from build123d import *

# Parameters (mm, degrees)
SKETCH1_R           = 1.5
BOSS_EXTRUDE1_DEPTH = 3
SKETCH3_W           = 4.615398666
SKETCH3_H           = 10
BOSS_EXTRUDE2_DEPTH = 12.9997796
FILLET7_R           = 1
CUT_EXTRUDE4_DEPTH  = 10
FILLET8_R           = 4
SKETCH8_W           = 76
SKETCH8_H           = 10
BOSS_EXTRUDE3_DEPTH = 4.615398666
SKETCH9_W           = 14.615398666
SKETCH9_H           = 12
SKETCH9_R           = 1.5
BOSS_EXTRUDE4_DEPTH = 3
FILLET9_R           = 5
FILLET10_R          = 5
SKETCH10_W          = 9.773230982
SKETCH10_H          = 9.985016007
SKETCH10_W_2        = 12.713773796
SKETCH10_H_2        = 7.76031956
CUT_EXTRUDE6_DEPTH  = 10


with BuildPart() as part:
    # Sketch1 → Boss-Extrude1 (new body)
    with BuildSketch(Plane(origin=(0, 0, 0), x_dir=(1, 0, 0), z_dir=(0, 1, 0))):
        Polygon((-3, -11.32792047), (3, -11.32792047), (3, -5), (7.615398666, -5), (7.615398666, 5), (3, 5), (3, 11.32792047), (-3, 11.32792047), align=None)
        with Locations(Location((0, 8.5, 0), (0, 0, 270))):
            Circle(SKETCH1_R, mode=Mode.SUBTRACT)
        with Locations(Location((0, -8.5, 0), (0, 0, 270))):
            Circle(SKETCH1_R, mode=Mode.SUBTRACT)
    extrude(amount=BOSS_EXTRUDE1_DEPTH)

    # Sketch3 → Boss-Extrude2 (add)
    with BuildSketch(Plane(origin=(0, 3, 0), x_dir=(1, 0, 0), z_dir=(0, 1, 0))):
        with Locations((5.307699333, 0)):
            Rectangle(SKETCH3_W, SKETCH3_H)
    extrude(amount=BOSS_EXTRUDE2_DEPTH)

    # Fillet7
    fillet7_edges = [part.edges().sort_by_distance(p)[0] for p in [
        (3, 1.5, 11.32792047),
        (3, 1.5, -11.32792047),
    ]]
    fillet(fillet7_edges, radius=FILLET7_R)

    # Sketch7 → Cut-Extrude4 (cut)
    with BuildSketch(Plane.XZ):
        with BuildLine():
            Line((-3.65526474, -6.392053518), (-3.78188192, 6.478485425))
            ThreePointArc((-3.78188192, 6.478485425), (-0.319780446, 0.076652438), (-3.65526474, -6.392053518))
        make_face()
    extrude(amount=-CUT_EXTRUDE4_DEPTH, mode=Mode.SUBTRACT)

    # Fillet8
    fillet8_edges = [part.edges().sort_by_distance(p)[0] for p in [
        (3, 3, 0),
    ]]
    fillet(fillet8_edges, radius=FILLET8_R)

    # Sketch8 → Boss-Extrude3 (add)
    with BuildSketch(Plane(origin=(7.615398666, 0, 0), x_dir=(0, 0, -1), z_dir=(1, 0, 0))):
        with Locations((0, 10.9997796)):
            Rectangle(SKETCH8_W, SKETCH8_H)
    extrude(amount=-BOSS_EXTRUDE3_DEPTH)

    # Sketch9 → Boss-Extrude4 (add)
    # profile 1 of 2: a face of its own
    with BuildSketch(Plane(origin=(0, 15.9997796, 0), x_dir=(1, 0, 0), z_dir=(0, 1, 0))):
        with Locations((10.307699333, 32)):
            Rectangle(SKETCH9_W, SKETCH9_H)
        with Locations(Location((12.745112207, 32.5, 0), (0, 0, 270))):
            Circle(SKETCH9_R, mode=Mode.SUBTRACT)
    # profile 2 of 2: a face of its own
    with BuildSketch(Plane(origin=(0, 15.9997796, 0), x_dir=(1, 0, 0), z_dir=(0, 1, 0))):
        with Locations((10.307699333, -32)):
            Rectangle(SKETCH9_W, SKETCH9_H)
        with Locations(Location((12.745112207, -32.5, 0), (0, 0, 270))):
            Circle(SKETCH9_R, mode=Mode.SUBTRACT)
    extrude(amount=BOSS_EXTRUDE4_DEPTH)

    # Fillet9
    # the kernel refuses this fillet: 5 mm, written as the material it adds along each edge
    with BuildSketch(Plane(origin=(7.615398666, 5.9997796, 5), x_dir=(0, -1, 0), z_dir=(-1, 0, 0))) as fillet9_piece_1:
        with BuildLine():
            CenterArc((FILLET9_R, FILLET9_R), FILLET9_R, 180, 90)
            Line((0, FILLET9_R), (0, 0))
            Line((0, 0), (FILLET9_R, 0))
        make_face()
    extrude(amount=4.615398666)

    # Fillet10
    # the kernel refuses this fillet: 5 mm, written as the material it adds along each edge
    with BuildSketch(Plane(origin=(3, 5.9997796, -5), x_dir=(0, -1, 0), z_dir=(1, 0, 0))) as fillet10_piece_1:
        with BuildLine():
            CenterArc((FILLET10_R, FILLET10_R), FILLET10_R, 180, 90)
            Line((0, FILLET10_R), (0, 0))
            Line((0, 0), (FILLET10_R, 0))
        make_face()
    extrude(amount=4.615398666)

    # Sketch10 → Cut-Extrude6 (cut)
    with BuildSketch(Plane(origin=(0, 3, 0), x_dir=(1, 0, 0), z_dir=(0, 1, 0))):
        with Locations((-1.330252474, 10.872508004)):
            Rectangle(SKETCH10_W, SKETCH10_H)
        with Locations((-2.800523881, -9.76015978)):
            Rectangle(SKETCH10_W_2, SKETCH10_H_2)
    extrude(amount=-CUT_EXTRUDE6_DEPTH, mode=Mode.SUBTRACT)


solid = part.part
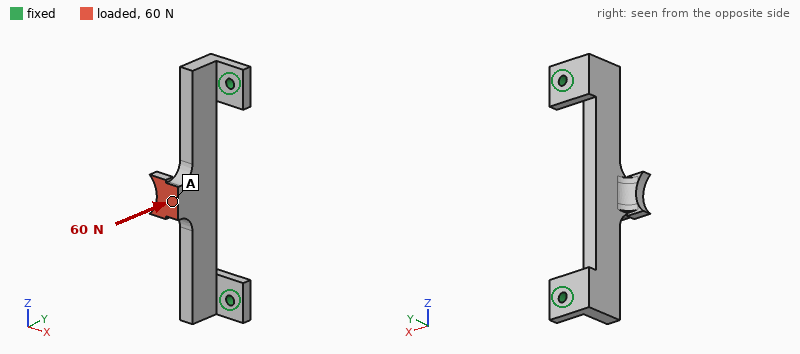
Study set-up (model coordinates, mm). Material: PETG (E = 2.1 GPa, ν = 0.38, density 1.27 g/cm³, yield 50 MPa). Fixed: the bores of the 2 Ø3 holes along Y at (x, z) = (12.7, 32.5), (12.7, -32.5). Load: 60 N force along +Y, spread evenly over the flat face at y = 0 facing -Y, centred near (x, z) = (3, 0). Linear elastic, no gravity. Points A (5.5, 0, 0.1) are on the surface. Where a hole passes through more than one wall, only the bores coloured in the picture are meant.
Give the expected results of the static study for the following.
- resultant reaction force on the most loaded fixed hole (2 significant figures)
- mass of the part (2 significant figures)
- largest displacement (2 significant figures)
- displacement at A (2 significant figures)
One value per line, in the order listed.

44 N
6.4 g
0.83 mm
0.65 mm
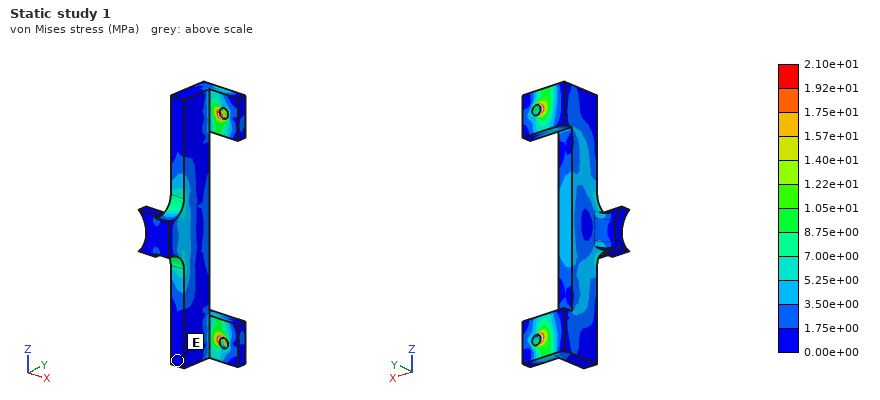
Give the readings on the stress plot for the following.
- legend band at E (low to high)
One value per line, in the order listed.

0.00e+00 to 1.75e+00 MPa
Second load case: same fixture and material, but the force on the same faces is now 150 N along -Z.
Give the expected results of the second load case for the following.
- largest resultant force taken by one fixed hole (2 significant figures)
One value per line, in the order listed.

86 N
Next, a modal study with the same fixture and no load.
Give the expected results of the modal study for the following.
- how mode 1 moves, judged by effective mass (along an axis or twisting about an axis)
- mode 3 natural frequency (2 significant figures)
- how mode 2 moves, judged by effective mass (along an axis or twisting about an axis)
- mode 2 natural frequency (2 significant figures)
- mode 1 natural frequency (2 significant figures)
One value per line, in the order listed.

along X
2000 Hz
along Y
1700 Hz
750 Hz
